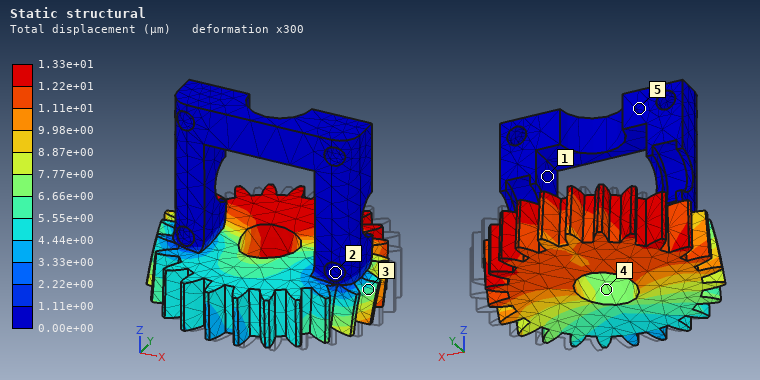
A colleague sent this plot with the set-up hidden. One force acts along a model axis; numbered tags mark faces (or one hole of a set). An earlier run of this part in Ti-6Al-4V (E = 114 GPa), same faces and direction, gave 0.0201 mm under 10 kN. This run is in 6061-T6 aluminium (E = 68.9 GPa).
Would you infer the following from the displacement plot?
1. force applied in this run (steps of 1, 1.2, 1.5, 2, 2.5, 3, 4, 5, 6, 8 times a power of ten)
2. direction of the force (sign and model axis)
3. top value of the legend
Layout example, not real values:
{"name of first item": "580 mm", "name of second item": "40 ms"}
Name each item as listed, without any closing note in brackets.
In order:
{"force applied in this run": "4 kN", "direction of the force": "-X", "top value of the legend": "1.33e+01 µm"}
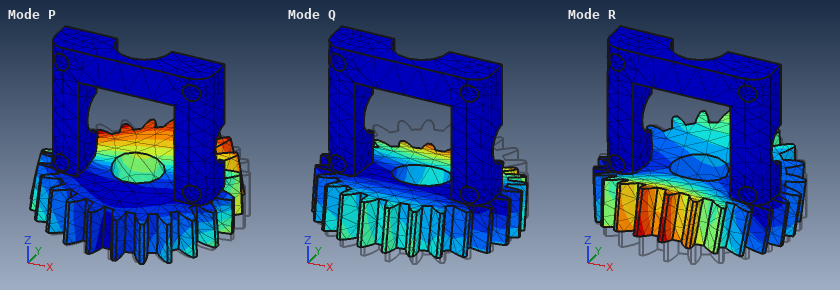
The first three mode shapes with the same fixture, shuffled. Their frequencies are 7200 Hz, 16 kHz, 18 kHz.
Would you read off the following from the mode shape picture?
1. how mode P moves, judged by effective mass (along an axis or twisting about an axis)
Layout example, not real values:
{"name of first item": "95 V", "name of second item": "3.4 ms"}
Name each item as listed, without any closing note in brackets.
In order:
{"how mode P moves, judged by effective mass": "along X"}
